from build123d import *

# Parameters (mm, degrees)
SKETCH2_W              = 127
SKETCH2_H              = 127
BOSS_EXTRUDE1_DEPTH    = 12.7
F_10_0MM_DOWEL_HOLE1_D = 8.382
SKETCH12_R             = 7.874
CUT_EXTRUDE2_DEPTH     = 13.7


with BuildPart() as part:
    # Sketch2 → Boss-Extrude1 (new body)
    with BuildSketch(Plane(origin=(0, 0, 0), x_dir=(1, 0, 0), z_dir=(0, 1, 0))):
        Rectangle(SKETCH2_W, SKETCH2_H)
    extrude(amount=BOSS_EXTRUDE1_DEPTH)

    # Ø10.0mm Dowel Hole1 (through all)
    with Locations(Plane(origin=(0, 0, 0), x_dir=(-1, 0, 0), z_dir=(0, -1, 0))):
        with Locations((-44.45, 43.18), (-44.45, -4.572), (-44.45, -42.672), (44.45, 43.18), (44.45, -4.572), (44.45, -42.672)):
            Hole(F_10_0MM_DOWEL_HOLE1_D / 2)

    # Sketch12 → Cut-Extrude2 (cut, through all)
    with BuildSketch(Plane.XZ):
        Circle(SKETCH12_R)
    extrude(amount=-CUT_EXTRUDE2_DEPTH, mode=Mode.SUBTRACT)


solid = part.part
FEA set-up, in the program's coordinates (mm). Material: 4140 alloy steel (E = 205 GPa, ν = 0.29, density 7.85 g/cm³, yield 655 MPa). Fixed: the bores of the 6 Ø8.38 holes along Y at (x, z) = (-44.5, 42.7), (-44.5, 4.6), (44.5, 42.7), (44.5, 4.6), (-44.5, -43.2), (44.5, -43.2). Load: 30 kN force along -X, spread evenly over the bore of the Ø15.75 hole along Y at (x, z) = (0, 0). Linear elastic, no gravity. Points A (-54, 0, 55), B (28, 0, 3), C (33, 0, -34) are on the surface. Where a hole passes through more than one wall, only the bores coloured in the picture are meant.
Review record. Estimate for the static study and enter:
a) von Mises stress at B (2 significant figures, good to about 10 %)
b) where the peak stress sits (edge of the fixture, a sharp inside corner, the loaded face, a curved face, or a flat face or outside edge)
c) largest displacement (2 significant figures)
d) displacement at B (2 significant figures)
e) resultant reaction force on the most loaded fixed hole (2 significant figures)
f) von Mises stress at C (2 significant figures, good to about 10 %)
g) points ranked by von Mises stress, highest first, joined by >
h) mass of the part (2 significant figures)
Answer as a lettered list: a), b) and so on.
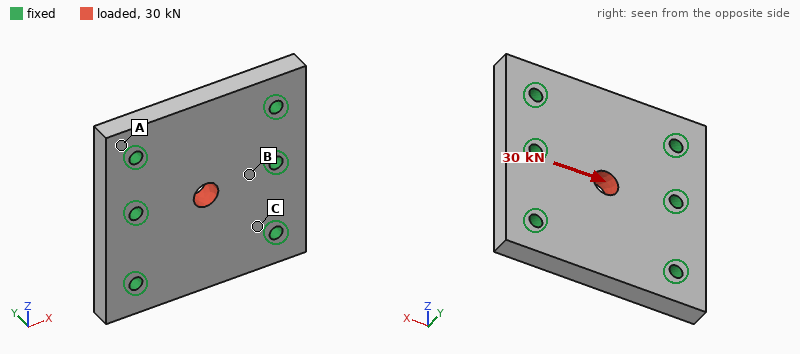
a) 31 MPa
b) the loaded face
c) 6.1 µm
d) 2.1 µm
e) 8.3 kN
f) 14 MPa
g) B > C > A
h) 1.6 kg
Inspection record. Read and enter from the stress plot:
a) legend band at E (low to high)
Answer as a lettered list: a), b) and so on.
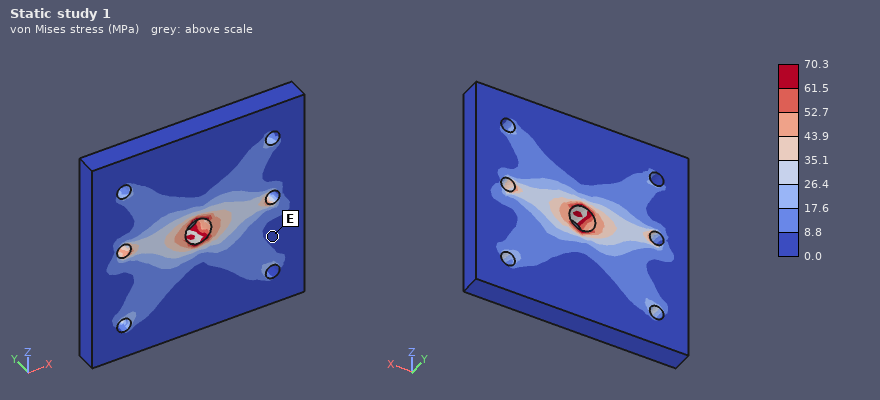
a) 0.0 to 8.8 MPa
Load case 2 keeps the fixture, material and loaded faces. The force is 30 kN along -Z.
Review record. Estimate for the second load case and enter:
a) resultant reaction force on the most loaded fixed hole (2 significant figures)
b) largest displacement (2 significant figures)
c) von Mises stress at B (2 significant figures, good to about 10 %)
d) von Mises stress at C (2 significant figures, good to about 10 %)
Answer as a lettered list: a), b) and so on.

a) 5.8 kN
b) 8.3 µm
c) 17 MPa
d) 22 MPa
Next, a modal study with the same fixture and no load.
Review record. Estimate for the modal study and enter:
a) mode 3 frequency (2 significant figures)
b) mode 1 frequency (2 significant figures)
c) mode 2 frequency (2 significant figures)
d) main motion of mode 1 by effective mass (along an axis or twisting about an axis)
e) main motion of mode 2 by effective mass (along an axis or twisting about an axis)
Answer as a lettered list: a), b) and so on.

a) 9800 Hz
b) 7100 Hz
c) 7600 Hz
d) along Y
e) twisting about X
